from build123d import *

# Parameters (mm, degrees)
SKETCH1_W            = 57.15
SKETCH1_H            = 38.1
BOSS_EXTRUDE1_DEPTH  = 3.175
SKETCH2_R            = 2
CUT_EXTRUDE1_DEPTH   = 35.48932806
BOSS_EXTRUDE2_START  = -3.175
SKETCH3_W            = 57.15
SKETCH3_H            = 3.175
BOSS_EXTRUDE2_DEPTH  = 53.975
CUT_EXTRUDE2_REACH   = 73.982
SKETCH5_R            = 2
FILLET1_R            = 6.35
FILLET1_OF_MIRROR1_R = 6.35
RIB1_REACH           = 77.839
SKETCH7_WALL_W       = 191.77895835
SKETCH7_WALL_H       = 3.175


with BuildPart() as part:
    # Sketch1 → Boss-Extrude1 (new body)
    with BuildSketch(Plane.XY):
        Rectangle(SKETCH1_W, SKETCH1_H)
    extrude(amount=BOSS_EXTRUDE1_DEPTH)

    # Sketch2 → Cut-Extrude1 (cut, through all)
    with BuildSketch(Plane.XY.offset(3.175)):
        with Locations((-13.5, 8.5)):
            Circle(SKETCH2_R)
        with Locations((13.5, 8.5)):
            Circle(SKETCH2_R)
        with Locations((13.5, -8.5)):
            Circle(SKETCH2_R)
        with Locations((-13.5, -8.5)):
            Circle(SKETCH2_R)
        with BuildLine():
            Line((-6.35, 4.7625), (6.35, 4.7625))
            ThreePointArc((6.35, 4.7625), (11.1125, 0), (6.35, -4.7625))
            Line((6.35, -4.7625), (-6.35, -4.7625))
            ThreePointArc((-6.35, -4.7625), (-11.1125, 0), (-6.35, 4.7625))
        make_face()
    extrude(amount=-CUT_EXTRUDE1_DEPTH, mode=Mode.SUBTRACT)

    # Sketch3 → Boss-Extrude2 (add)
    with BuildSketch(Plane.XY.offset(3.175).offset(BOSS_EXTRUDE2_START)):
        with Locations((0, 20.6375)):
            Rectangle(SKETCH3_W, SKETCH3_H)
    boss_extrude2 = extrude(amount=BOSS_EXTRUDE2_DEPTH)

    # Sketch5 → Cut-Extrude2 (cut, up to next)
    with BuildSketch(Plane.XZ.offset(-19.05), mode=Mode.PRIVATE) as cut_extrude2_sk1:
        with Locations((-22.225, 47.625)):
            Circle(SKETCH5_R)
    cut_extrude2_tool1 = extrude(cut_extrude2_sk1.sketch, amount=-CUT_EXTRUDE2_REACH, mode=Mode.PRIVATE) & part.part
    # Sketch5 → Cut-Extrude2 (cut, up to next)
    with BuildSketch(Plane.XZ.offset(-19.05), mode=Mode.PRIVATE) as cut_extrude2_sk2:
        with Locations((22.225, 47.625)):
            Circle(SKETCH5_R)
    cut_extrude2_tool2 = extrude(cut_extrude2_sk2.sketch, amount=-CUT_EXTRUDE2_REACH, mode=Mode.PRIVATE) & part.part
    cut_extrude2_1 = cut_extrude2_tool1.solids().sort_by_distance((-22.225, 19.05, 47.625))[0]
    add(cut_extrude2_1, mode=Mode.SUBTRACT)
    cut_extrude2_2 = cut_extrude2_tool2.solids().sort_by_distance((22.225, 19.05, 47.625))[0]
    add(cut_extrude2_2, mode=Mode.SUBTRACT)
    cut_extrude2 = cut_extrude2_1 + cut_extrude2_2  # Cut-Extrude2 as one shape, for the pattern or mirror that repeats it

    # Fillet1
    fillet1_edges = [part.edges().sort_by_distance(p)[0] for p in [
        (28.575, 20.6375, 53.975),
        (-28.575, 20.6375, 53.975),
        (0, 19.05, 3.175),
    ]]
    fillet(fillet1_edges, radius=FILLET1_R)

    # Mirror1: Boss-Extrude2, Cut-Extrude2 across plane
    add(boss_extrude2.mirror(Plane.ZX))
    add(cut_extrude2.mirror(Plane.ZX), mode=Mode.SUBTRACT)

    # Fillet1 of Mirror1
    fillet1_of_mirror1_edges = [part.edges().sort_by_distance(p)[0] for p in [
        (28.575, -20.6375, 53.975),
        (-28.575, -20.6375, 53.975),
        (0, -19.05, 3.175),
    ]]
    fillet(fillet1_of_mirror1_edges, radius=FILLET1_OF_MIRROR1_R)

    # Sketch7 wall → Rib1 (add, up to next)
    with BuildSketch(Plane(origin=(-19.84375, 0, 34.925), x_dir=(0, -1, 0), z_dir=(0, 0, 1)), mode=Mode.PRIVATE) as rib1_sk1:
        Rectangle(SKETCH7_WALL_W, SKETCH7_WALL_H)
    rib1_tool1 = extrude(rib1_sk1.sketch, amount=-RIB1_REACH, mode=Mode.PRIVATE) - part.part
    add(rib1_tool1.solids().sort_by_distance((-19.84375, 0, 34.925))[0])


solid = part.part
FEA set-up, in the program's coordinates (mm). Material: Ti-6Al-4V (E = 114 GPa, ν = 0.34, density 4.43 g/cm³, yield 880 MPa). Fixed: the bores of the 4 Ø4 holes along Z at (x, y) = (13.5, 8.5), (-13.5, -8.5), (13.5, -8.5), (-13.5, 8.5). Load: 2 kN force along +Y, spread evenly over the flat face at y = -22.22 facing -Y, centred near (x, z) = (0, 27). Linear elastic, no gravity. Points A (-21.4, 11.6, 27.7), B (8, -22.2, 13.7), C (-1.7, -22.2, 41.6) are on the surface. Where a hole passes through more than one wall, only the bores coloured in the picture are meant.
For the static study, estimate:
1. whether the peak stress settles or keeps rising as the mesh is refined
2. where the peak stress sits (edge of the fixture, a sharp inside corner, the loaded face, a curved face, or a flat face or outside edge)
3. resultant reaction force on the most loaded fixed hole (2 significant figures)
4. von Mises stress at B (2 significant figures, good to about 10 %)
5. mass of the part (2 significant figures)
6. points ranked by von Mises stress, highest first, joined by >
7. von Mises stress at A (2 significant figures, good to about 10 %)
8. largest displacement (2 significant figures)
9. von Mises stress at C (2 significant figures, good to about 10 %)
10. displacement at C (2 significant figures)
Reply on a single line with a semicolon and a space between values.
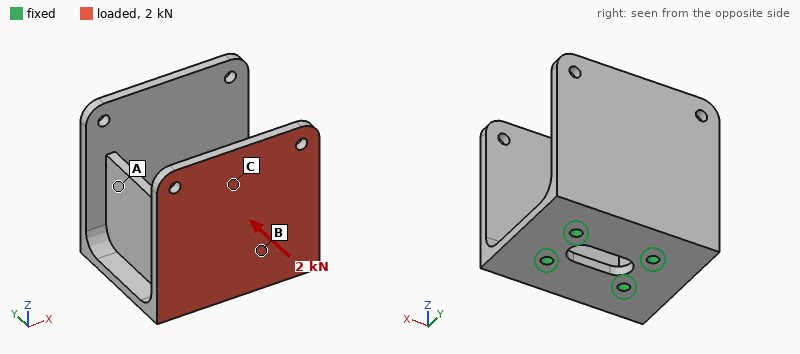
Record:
keeps rising; edge of the fixture; 2.2 kN; 110 MPa; 130 g; B > C > A; 32 MPa; 0.99 mm; 71 MPa; 0.41 mm
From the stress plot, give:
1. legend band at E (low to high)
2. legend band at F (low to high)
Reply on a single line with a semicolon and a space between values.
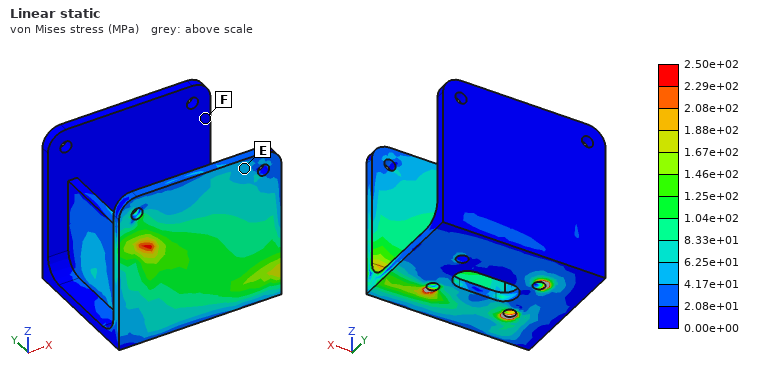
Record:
4.17e+01 to 6.25e+01 MPa; 0.00e+00 to 2.08e+01 MPa
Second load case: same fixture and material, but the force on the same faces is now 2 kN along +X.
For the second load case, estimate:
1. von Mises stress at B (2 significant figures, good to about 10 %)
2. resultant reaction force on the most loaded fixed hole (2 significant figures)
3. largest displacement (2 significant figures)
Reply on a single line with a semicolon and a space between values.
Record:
30 MPa; 2.1 kN; 0.16 mm
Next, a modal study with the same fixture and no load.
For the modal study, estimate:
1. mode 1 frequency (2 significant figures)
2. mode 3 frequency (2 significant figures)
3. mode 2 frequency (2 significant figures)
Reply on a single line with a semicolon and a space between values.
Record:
1500 Hz; 2600 Hz; 1500 Hz
